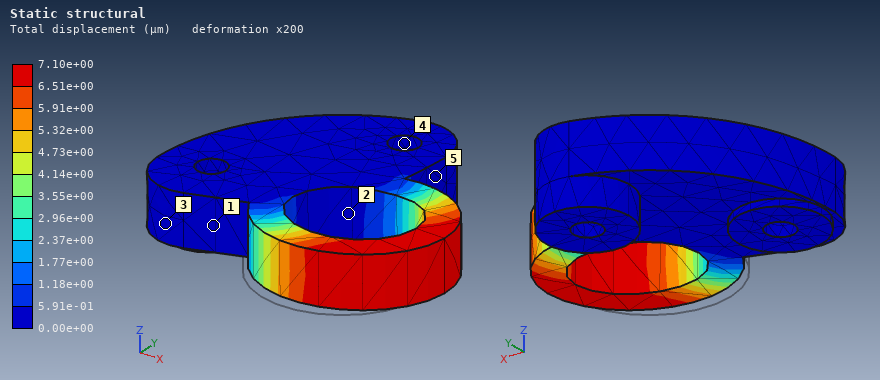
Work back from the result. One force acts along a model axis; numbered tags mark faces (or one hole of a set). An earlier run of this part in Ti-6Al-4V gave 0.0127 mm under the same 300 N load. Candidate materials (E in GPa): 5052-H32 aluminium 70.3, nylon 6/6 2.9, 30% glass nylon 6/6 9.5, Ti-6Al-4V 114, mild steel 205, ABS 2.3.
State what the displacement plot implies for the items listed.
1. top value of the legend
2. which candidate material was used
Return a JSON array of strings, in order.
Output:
["7.10e+00 µm", "mild steel"]
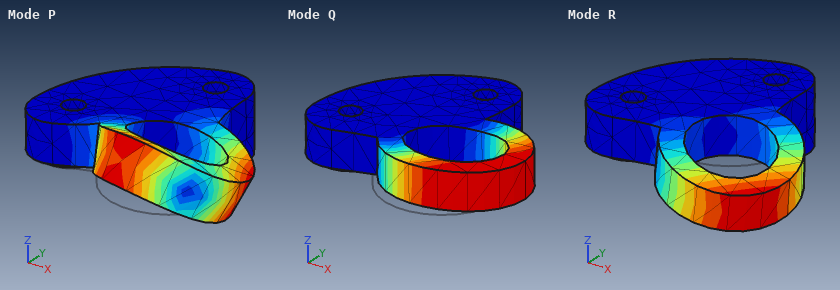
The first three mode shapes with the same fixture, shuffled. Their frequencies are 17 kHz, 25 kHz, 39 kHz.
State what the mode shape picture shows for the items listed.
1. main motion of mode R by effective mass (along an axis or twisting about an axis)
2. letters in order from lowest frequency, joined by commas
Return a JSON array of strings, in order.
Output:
["along Z", "R, Q, P"]
